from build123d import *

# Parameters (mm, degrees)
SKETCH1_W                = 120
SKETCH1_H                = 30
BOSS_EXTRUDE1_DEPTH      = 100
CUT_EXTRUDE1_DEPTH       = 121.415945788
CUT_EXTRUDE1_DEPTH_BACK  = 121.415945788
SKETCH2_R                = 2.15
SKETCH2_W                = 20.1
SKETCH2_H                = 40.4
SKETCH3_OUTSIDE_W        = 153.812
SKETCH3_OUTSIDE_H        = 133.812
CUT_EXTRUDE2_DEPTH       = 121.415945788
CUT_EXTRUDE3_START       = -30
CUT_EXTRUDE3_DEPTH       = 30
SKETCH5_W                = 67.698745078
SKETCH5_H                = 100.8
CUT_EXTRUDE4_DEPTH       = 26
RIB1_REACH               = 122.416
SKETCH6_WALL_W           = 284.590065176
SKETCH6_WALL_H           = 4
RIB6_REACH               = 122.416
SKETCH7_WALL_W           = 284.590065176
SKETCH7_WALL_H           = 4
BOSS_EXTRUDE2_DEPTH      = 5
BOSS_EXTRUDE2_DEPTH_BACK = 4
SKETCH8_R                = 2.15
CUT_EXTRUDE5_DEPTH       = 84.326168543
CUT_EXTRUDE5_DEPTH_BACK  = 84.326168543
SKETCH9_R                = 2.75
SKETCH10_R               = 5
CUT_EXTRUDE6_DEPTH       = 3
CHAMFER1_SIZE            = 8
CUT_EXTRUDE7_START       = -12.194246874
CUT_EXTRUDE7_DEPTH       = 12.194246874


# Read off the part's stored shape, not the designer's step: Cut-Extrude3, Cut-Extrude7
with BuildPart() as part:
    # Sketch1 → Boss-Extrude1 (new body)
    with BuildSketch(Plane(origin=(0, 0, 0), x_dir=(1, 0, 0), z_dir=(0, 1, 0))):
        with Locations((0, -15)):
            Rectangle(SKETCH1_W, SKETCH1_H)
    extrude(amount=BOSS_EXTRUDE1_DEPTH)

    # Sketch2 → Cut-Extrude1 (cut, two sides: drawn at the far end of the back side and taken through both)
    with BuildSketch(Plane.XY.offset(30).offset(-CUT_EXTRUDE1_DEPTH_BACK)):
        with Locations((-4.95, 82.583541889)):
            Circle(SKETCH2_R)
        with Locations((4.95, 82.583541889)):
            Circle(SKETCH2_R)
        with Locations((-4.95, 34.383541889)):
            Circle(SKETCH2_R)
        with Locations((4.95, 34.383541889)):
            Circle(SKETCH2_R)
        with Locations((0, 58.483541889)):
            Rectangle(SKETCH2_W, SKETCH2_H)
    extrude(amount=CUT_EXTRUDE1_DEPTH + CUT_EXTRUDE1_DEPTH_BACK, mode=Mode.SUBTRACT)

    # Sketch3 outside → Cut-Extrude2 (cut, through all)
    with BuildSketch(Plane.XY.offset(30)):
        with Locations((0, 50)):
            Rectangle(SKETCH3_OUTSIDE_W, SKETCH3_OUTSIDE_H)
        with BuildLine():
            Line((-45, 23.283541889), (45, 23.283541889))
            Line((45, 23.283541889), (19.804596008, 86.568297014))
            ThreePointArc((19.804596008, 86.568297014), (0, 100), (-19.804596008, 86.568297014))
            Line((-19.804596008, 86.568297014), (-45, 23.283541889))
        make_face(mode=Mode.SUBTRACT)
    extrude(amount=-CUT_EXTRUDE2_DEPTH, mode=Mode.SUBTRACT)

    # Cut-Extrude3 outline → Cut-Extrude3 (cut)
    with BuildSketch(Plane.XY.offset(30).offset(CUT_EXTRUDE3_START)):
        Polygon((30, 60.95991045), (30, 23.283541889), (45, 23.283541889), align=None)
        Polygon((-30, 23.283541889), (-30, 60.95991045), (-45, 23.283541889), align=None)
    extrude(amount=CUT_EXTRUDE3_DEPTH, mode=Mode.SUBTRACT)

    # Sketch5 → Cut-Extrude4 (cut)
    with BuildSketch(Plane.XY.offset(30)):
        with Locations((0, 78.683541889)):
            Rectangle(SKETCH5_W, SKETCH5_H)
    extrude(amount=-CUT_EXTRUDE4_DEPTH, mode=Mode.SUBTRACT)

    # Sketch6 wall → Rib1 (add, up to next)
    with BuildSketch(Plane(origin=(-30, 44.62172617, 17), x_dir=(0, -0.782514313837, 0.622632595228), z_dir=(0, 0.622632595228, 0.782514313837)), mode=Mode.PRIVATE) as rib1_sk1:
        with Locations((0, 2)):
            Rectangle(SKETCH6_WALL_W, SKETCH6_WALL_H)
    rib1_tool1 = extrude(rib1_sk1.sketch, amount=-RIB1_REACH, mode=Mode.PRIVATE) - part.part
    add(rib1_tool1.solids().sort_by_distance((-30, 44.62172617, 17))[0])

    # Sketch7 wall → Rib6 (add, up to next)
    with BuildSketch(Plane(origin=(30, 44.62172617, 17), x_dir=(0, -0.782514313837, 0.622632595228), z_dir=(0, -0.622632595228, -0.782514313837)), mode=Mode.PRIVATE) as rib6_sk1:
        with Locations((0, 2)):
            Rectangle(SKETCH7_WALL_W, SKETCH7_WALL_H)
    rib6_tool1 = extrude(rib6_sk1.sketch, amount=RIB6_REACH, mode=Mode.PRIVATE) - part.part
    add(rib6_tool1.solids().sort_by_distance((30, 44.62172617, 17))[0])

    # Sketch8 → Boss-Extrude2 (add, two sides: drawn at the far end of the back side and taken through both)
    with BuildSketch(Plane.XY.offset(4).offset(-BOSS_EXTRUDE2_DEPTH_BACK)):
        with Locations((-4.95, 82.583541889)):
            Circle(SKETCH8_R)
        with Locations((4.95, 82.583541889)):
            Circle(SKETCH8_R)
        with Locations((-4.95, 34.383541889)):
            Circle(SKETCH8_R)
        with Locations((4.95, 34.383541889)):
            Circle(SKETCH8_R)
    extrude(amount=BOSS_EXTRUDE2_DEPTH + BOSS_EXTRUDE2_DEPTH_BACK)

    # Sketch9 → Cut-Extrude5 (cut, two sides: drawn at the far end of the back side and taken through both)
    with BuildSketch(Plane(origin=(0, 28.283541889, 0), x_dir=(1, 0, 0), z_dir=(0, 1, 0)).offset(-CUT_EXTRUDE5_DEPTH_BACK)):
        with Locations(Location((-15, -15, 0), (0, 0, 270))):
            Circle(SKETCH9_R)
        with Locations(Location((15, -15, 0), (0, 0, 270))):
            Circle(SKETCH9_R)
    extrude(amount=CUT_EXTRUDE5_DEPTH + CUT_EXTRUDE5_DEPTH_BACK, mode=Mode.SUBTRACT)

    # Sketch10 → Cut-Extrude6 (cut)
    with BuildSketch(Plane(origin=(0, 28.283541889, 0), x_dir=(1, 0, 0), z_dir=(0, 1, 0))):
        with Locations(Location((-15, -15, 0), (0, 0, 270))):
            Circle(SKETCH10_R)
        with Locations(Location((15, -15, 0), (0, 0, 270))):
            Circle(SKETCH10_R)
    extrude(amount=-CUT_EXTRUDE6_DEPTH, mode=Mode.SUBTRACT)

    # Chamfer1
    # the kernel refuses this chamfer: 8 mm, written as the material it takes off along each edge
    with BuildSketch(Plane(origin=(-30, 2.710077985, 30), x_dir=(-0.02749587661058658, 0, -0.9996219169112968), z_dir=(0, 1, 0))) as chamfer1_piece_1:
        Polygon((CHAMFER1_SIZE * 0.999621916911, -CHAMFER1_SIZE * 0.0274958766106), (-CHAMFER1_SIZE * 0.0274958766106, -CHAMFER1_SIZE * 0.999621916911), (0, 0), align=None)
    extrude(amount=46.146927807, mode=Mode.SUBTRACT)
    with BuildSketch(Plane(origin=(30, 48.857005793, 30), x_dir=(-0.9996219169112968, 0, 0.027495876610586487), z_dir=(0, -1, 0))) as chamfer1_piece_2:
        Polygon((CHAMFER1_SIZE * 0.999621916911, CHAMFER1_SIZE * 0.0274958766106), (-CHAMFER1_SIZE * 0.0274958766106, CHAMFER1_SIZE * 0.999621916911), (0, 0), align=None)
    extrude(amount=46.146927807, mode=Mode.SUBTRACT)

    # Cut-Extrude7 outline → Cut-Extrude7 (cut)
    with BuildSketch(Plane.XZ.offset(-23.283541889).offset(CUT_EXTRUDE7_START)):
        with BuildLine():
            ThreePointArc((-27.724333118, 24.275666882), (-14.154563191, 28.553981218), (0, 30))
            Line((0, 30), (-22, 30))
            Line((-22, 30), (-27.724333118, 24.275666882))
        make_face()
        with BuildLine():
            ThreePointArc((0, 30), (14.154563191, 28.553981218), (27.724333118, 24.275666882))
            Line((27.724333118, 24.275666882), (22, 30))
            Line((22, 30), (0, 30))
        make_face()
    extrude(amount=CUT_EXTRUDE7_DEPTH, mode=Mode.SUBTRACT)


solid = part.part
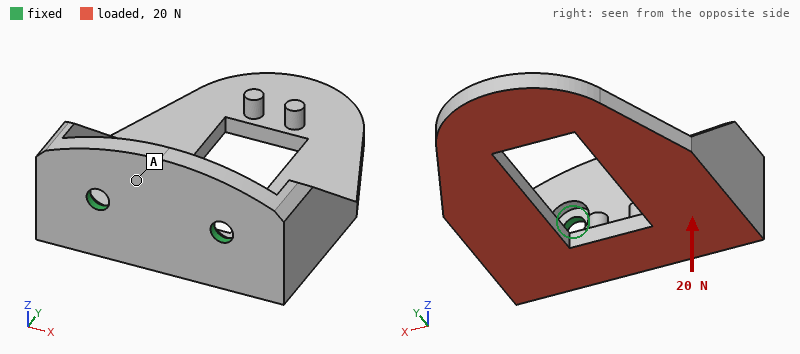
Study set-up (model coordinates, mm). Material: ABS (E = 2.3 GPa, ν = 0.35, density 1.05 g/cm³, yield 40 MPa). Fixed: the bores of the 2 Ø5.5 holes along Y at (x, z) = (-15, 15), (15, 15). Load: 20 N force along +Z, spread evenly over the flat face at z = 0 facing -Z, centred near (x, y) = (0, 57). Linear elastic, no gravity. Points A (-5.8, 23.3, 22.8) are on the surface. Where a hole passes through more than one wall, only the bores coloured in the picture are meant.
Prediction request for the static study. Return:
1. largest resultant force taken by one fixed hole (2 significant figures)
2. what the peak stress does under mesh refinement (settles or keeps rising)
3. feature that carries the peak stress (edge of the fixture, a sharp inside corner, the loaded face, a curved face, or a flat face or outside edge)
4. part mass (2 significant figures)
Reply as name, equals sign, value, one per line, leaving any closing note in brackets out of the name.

largest resultant force taken by one fixed hole = 16 N
what the peak stress does under mesh refinement = keeps rising
feature that carries the peak stress = edge of the fixture
part mass = 24 g
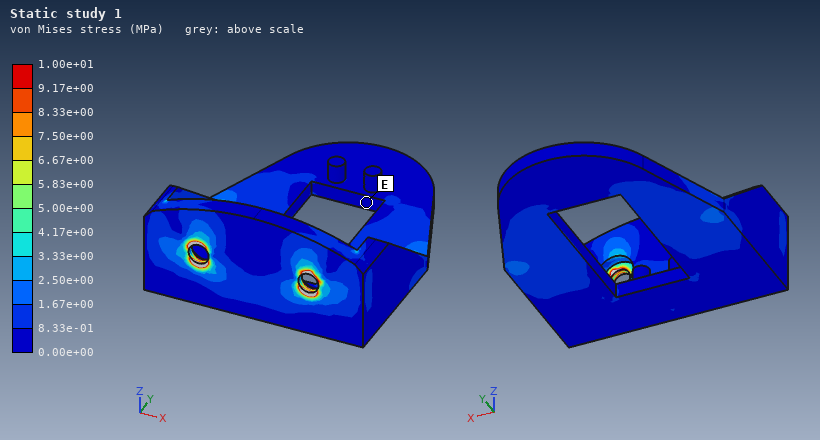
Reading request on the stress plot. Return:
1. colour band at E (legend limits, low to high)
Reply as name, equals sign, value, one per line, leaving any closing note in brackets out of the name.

colour band at E = 0.00e+00 to 8.33e-01 MPa
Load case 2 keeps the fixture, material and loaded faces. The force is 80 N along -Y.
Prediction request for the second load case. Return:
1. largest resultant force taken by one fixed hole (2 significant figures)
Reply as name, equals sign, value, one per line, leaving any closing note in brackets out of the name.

largest resultant force taken by one fixed hole = 40 N
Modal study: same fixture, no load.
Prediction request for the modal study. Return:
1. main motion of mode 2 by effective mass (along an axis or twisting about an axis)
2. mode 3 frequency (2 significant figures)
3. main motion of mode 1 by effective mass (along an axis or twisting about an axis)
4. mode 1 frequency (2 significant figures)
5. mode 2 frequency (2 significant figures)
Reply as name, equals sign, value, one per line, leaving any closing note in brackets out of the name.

main motion of mode 2 by effective mass = along X
mode 3 frequency = 850 Hz
main motion of mode 1 by effective mass = along Z
mode 1 frequency = 240 Hz
mode 2 frequency = 520 Hz
